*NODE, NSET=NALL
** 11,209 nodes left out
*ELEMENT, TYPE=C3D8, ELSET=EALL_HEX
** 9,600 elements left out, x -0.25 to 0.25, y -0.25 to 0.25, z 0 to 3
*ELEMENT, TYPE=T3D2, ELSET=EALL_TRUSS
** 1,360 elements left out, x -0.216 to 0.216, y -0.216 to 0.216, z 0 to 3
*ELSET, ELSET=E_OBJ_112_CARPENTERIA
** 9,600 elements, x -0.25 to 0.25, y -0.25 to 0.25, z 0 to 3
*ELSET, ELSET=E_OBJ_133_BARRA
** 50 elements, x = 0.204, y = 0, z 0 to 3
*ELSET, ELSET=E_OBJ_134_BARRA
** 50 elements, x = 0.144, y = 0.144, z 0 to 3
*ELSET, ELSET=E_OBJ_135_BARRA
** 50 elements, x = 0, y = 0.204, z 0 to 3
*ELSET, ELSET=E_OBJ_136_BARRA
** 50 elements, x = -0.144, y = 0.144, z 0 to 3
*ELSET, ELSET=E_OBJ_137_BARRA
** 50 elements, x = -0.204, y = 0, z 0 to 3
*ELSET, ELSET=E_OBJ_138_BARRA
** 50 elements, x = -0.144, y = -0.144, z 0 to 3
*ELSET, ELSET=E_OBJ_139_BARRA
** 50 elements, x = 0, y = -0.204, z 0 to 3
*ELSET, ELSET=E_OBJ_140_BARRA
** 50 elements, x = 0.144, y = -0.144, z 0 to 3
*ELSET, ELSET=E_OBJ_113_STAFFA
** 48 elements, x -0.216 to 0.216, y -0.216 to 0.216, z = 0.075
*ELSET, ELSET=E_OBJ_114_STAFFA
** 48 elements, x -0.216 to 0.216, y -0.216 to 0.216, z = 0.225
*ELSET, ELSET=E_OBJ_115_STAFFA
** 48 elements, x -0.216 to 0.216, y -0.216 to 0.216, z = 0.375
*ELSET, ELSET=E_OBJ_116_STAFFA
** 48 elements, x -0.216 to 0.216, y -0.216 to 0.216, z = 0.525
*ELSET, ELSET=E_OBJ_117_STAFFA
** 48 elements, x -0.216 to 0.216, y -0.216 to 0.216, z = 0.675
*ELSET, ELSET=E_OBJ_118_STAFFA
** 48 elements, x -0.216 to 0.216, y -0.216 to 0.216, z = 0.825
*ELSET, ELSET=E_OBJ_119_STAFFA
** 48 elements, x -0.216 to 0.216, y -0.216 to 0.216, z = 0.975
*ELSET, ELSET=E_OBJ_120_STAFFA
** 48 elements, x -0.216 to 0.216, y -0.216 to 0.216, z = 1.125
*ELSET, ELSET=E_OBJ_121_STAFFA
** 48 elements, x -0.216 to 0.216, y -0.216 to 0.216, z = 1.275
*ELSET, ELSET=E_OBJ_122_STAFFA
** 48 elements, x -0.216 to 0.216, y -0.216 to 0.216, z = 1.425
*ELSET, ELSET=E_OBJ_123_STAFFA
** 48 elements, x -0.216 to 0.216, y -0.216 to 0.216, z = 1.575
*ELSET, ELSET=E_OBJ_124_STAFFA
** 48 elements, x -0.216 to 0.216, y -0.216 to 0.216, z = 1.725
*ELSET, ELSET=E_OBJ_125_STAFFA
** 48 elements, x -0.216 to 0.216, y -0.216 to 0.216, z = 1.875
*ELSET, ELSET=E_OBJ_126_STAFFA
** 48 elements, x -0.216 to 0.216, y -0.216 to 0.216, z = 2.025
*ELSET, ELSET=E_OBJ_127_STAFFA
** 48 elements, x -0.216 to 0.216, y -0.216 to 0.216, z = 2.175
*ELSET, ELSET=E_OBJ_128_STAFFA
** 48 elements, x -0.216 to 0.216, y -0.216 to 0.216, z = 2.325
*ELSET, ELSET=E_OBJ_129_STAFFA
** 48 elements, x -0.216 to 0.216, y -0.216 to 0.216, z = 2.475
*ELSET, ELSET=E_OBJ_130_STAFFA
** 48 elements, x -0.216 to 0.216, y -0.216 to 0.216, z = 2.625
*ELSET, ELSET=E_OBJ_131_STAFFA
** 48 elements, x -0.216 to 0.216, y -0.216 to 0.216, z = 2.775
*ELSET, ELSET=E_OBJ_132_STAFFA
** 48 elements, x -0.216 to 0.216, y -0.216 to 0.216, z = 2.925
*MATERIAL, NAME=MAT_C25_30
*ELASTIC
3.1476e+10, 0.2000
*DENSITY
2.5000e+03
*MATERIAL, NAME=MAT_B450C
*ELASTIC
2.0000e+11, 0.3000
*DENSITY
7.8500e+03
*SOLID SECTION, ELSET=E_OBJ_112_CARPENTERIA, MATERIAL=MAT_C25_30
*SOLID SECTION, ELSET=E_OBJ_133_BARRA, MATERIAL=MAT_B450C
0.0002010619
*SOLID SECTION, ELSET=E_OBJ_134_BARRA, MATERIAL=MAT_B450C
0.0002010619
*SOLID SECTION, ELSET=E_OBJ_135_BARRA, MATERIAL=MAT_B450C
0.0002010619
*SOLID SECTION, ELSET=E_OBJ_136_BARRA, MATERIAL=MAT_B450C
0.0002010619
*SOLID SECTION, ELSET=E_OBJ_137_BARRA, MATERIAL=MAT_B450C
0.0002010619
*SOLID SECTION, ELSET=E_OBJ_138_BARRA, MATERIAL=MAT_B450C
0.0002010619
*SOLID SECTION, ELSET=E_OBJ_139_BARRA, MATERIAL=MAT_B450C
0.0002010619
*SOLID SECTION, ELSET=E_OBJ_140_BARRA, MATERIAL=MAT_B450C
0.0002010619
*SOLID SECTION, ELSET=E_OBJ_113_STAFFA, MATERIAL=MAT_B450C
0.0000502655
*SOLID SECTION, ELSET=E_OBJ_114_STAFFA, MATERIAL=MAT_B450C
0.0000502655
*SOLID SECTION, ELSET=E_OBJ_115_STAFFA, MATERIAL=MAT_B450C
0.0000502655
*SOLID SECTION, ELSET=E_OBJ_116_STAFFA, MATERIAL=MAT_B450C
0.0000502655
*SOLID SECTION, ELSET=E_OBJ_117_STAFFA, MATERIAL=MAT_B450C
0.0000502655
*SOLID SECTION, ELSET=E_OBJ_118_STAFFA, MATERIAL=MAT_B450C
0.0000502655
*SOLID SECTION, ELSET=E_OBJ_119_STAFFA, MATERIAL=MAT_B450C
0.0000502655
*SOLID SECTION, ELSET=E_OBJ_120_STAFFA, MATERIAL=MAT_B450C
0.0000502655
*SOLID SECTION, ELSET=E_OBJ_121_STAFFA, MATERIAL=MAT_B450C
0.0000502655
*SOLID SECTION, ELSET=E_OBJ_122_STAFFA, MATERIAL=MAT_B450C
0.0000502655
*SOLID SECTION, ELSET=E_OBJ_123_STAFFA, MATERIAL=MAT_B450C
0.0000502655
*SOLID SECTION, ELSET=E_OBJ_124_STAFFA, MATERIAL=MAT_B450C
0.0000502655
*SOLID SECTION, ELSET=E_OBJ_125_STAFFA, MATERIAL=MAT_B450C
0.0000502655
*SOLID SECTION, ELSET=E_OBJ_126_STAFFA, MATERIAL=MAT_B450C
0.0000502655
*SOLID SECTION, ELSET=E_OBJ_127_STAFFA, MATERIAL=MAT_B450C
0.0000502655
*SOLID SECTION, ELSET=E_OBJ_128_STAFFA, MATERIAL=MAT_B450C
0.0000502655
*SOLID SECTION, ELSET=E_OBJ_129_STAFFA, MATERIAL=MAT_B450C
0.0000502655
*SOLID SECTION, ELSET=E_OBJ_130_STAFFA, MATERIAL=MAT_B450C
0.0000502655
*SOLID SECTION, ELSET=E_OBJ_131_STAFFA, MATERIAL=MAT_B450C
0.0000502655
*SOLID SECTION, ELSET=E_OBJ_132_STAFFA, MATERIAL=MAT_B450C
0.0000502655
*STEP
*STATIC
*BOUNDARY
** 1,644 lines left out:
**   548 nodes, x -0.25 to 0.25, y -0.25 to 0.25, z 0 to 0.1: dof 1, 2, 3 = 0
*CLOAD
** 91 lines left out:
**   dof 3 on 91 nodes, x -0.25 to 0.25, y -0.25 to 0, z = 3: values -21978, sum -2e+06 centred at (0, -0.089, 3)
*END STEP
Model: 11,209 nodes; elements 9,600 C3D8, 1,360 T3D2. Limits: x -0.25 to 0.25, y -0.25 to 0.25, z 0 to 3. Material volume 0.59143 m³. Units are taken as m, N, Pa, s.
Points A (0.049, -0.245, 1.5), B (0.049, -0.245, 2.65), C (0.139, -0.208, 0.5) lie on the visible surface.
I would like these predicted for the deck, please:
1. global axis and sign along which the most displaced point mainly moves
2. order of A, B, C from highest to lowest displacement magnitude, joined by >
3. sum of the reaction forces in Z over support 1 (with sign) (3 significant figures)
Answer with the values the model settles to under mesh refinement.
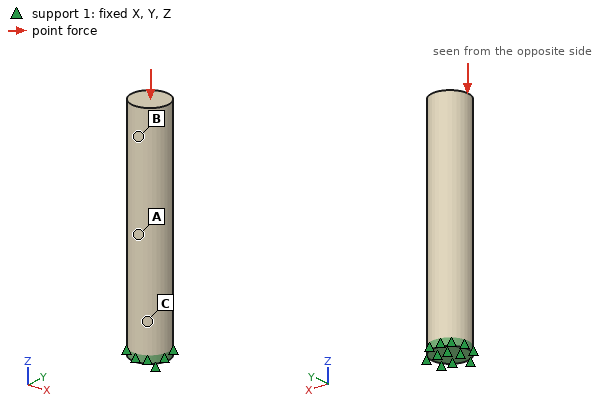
-X
B > A > C
2.00e+06 N
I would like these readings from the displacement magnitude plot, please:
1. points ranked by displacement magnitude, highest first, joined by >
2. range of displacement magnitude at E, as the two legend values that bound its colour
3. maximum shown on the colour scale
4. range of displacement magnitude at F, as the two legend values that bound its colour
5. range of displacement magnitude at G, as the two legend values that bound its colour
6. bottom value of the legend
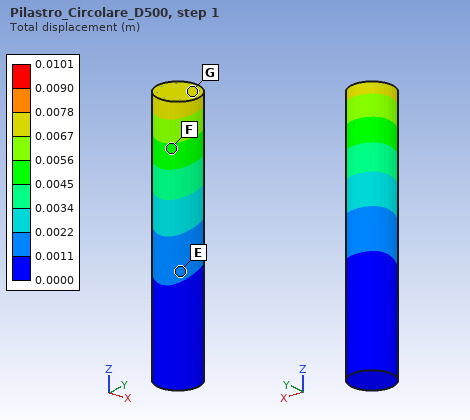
G > F > E
0.0011 to 0.0022 m
0.0101 m
0.0045 to 0.0056 m
0.0067 to 0.0078 m
0.0000 m
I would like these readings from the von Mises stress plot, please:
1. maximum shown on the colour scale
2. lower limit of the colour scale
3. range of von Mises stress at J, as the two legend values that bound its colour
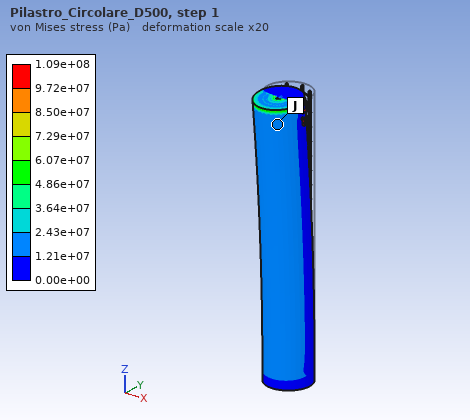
1.09e+08 Pa
0.00e+00 Pa
1.21e+07 to 2.43e+07 Pa
